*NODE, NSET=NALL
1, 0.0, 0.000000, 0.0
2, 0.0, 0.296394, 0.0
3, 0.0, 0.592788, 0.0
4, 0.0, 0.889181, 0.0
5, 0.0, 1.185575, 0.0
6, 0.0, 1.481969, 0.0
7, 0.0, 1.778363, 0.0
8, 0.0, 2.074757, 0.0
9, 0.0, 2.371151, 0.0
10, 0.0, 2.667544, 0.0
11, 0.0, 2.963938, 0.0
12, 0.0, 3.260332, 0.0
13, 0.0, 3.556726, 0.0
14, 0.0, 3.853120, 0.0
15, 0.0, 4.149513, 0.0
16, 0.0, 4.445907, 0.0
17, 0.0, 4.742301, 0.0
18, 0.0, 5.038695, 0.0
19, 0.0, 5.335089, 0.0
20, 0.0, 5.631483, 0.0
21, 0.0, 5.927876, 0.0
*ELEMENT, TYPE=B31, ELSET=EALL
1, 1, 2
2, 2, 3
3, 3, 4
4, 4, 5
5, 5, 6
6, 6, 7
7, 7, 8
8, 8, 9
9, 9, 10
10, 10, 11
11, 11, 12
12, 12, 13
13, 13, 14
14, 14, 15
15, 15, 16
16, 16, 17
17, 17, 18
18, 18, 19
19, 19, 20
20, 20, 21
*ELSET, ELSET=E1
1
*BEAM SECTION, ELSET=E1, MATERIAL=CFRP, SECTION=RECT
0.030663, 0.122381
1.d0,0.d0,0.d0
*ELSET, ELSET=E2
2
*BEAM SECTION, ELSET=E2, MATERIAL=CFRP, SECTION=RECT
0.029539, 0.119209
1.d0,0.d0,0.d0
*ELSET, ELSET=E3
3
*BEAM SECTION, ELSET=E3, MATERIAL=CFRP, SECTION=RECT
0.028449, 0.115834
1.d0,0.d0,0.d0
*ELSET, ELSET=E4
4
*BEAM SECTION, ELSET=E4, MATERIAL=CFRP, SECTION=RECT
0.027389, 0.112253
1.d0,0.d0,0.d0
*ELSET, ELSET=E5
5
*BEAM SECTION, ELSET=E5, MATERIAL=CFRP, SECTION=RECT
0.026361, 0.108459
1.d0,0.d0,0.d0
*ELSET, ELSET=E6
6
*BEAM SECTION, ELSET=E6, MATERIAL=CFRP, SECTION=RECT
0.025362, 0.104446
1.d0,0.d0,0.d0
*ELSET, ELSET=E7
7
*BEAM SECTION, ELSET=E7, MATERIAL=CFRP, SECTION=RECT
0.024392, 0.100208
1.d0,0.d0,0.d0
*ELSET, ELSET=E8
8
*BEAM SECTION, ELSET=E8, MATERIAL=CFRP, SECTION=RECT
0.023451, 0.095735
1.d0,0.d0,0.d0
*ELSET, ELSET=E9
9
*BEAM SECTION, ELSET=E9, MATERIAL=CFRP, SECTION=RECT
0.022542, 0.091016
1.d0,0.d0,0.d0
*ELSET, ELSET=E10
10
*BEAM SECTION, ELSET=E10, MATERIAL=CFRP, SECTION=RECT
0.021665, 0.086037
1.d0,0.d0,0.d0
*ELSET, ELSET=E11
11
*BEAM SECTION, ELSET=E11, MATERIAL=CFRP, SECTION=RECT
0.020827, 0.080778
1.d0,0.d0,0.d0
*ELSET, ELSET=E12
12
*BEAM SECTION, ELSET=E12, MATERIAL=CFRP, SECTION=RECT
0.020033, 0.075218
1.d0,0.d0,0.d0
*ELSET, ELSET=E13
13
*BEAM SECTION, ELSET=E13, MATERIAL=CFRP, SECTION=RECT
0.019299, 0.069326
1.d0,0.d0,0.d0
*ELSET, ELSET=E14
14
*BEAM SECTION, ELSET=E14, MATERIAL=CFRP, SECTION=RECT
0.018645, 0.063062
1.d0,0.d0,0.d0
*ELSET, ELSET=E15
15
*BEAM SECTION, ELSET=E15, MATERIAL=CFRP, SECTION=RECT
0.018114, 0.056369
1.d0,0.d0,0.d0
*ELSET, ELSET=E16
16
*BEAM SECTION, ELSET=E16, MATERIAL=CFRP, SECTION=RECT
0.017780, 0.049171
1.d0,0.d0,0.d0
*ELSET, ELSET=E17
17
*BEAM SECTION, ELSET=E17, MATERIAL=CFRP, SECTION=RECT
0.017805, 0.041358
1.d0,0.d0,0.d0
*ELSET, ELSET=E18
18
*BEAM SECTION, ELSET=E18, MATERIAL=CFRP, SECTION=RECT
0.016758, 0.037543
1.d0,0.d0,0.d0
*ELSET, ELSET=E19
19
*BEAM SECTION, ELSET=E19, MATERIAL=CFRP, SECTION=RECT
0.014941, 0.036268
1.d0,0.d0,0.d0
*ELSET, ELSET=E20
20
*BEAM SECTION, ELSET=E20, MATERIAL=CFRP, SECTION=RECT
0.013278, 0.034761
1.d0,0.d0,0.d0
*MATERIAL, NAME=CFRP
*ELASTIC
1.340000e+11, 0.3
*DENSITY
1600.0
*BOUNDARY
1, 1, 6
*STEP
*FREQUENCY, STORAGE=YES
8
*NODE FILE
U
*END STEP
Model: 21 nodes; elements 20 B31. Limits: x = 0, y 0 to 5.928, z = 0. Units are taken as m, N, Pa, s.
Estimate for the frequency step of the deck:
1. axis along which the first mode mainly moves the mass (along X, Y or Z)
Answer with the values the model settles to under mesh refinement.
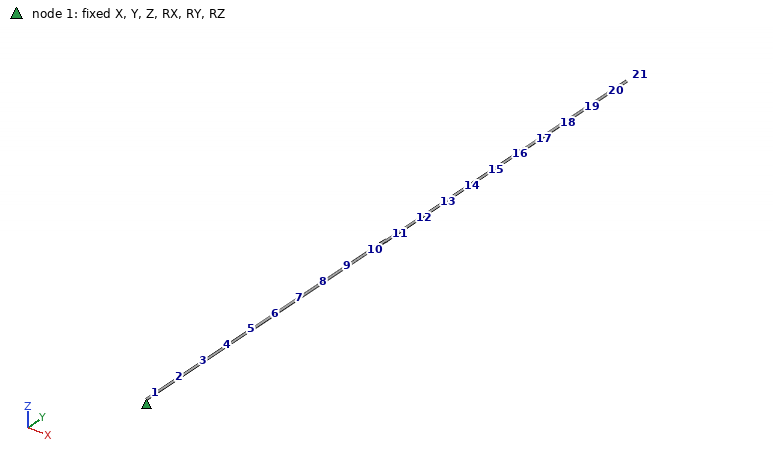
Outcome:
along X
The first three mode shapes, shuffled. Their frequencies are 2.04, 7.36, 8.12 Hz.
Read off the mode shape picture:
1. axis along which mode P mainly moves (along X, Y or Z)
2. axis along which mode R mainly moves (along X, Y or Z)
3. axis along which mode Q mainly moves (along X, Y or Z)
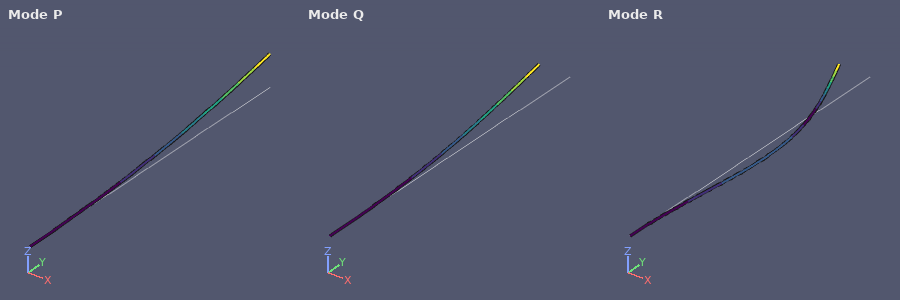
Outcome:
along Z
along X
along X
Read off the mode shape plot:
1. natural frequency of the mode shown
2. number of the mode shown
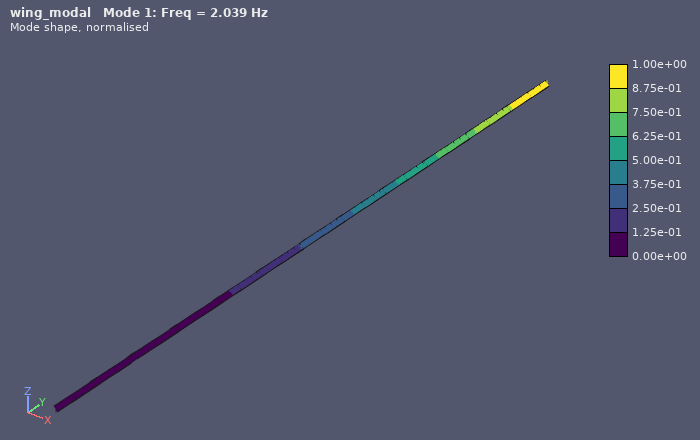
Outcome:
2.039 Hz
1
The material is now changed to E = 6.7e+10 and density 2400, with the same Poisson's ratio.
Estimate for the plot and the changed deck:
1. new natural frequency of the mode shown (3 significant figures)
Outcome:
1.18 Hz
